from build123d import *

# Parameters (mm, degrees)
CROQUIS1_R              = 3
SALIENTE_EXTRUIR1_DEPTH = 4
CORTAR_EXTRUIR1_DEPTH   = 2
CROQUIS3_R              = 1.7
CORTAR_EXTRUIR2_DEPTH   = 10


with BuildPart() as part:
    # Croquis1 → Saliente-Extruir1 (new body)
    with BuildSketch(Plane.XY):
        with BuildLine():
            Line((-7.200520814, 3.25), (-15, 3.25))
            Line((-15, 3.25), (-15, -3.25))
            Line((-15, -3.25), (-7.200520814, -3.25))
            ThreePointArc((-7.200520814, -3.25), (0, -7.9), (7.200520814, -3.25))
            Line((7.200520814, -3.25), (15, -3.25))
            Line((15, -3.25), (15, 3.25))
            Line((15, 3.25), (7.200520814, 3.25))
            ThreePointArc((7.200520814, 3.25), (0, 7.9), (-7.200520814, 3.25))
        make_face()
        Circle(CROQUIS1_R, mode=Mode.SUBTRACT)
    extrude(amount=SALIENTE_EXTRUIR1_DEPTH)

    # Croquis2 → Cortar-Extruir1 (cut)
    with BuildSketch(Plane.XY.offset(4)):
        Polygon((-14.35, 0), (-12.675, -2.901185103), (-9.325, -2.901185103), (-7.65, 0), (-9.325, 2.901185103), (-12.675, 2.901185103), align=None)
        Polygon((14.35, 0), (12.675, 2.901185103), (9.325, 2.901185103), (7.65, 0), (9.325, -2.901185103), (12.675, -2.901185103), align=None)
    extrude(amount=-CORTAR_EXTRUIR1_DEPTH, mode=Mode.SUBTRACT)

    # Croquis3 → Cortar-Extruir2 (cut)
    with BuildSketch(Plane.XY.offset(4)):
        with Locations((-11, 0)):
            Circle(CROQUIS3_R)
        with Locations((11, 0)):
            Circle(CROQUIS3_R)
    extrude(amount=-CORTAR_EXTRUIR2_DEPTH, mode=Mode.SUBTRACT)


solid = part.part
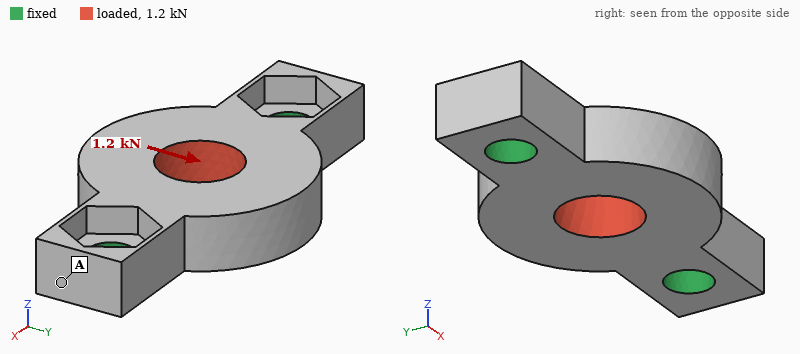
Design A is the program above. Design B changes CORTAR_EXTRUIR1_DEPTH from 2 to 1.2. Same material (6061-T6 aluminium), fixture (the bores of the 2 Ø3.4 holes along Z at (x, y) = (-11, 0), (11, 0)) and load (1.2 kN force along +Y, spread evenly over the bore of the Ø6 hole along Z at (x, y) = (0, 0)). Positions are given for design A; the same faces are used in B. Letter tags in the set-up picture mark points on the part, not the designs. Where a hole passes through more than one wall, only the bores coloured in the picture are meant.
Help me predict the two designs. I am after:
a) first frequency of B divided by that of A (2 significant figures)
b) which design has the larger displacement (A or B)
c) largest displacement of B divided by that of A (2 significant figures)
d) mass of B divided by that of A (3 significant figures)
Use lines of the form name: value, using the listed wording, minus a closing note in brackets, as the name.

first frequency of B divided by that of A: 1.2
which design has the larger displacement: A
largest displacement of B divided by that of A: 0.52
mass of B divided by that of A: 1.04
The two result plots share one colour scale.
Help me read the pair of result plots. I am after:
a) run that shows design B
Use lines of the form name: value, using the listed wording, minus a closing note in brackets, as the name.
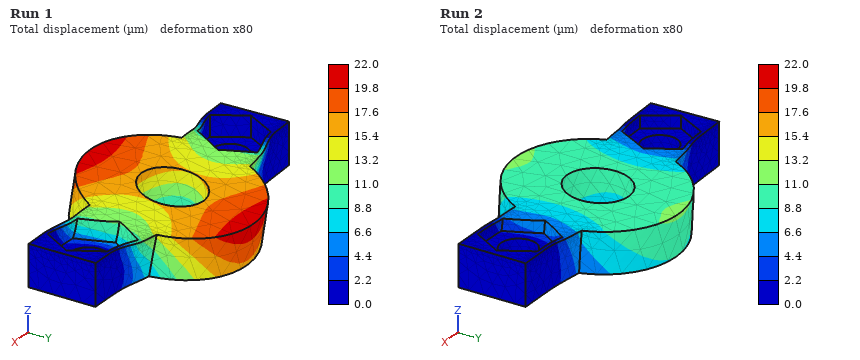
run that shows design B: Run 2
